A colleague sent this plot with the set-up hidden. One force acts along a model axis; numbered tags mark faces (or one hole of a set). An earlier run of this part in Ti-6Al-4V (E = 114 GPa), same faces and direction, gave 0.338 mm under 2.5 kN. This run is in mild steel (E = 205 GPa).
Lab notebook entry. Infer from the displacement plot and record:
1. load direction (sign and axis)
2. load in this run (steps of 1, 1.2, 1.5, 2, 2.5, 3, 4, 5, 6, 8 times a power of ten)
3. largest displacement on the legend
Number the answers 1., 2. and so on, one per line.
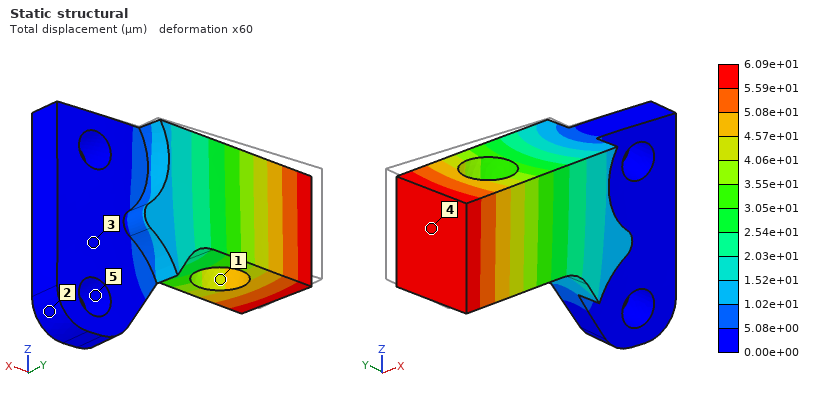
1. -Y
2. 800 N
3. 6.09e+01 µm
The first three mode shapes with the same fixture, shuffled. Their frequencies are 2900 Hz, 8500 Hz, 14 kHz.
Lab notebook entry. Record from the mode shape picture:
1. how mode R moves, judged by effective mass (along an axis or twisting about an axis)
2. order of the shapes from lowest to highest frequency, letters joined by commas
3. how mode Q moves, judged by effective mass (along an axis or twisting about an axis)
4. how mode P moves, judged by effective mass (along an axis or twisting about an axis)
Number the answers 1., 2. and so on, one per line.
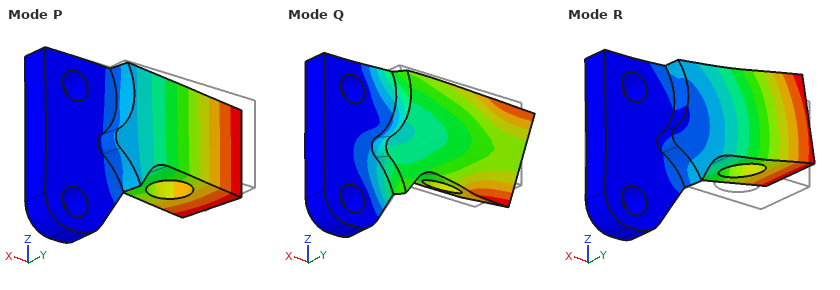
1. along Z
2. P, R, Q
3. twisting about X
4. along Y
